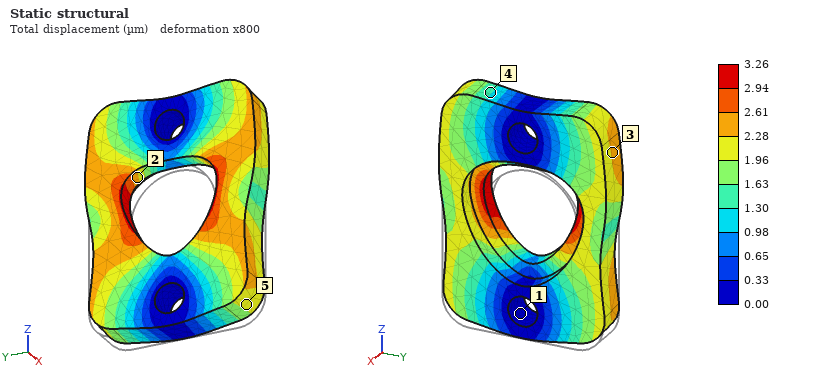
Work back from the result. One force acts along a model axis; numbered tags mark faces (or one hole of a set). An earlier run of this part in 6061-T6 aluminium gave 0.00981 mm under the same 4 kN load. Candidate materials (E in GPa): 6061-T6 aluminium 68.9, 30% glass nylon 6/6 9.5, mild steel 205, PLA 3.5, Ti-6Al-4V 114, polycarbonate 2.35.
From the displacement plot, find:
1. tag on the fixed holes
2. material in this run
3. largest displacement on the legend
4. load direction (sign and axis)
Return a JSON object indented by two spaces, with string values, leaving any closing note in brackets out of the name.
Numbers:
{
  "tag on the fixed holes": "1",
  "material in this run": "mild steel",
  "largest displacement on the legend": "3.26 µm",
  "load direction": "+Z"
}
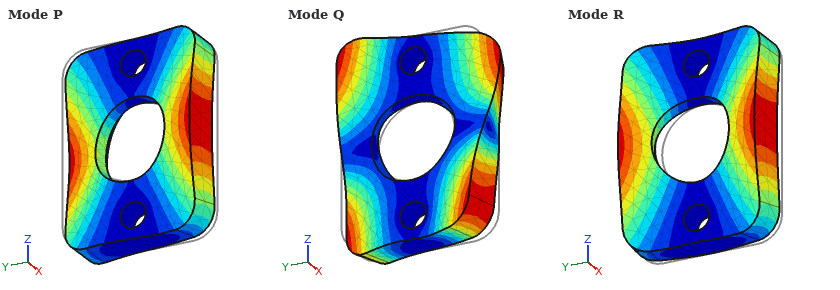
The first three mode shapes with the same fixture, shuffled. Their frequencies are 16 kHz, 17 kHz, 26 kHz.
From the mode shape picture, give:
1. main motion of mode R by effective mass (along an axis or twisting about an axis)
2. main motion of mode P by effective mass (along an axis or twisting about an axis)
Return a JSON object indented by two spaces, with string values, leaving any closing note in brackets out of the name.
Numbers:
{
  "main motion of mode R by effective mass": "along X",
  "main motion of mode P by effective mass": "twisting about Z"
}
